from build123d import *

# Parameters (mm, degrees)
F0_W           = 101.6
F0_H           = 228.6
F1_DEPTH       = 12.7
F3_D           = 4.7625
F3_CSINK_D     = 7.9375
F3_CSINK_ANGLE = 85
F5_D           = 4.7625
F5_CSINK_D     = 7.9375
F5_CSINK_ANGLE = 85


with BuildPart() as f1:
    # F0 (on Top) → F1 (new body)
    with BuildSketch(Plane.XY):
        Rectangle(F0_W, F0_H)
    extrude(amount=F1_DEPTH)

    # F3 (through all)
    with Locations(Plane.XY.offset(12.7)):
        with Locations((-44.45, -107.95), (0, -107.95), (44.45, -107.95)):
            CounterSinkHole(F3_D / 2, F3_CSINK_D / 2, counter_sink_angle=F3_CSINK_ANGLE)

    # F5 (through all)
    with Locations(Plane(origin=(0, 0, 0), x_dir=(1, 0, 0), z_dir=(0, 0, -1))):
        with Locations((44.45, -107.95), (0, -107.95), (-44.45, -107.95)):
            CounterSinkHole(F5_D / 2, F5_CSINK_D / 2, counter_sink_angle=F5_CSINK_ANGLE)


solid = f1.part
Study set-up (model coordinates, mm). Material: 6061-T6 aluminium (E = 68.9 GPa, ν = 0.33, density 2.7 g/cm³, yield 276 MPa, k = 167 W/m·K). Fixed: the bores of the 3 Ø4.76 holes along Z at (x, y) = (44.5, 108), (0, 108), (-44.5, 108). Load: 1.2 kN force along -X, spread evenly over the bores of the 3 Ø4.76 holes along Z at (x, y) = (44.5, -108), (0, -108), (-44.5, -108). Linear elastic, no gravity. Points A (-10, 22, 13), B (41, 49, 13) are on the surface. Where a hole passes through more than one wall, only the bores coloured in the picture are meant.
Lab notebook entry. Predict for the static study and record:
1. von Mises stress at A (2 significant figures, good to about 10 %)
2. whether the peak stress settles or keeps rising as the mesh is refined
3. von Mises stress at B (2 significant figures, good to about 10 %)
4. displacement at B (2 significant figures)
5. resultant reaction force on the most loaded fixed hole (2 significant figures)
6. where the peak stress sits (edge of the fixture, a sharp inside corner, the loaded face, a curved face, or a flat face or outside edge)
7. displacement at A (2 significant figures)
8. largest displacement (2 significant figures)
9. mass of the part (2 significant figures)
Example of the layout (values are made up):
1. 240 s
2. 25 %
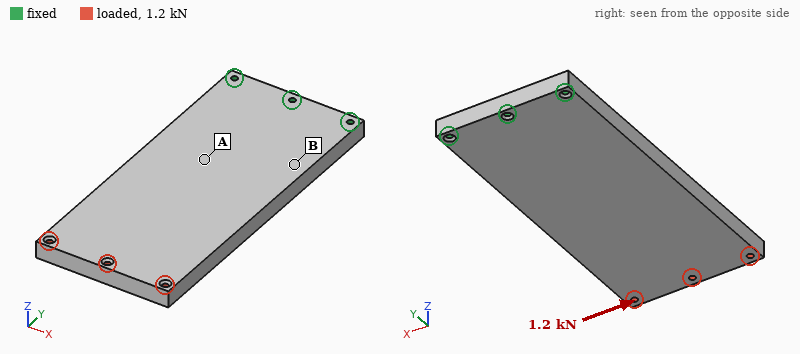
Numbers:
1. 2.5 MPa
2. keeps rising
3. 7.0 MPa
4. 13 µm
5. 3.0 kN
6. edge of the fixture
7. 17 µm
8. 75 µm
9. 790 g
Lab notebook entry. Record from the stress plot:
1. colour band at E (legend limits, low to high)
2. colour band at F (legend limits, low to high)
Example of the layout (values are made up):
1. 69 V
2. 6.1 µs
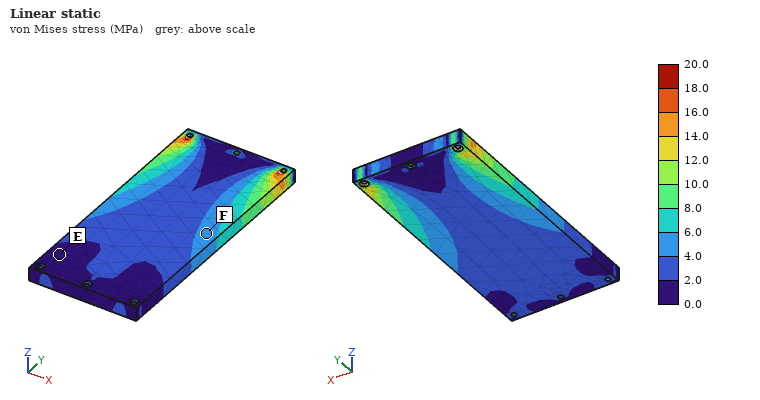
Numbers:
1. 0.0 to 2.0 MPa
2. 4.0 to 6.0 MPa
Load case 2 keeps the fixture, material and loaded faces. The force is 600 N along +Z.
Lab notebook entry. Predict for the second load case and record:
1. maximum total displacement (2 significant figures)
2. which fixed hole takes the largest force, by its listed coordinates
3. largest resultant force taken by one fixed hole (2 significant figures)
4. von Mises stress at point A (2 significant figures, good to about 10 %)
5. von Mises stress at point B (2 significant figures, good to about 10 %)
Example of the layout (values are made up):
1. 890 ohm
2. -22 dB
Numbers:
1. 2.0 mm
2. (0, 108)
3. 840 N
4. 28 MPa
5. 35 MPa
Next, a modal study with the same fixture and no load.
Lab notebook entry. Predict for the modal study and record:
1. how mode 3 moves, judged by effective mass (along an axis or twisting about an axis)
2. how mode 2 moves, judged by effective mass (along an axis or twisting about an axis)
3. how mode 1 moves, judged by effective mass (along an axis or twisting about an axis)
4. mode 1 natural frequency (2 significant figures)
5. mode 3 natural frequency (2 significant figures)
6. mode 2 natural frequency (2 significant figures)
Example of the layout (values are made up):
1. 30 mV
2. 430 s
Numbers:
1. along Z
2. twisting about Y
3. along Z
4. 190 Hz
5. 1200 Hz
6. 920 Hz
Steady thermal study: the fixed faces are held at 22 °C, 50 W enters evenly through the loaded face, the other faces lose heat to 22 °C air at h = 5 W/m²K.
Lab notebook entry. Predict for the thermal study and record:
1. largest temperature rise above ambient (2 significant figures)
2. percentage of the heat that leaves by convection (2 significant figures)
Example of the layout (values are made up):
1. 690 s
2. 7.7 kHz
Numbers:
1. 51 K
2. 13 %
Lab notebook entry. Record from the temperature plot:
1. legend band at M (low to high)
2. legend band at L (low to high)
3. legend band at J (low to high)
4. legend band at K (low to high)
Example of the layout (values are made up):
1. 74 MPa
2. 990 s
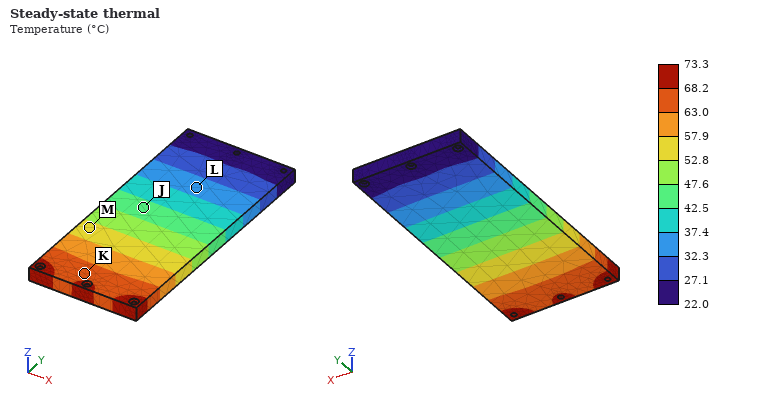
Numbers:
1. 52.8 to 57.9 °C
2. 32.3 to 37.4 °C
3. 42.5 to 47.6 °C
4. 63.0 to 68.2 °C
